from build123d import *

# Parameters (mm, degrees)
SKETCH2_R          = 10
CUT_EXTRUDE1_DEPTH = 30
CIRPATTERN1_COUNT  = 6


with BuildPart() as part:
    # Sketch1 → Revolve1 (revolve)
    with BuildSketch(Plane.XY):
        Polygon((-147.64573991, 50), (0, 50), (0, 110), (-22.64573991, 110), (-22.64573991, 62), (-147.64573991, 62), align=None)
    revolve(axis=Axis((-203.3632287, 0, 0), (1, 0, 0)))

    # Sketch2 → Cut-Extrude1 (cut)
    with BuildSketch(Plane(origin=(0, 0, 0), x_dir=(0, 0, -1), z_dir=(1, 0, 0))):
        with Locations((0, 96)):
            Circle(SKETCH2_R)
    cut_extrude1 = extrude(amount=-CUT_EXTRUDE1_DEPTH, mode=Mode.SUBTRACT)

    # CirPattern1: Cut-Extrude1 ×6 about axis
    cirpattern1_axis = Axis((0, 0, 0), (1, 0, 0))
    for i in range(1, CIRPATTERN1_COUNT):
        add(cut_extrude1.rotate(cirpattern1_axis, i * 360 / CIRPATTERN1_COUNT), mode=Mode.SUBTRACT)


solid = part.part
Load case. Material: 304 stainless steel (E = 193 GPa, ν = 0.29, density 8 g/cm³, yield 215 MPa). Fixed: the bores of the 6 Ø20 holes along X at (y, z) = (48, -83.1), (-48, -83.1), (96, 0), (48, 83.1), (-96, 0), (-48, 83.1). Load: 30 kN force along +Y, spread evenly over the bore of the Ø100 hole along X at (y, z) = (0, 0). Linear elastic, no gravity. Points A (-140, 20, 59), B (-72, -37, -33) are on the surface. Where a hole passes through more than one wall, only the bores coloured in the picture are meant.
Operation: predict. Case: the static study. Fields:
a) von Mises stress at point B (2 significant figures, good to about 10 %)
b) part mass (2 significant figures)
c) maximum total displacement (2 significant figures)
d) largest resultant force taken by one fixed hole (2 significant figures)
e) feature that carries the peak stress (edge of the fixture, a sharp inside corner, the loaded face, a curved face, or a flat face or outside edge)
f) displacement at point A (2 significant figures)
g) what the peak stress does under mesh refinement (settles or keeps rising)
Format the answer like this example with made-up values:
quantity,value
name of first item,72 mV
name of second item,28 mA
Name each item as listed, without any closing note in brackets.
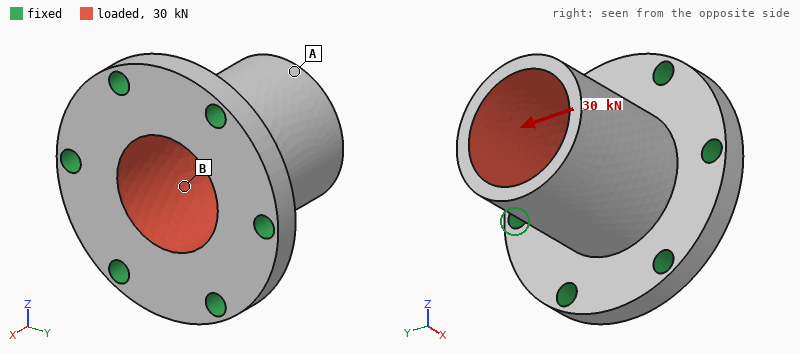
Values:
quantity,value
von Mises stress at point B,12 MPa
part mass,9.3 kg
maximum total displacement,33 µm
largest resultant force taken by one fixed hole,11 kN
feature that carries the peak stress,edge of the fixture
displacement at point A,29 µm
what the peak stress does under mesh refinement,keeps rising
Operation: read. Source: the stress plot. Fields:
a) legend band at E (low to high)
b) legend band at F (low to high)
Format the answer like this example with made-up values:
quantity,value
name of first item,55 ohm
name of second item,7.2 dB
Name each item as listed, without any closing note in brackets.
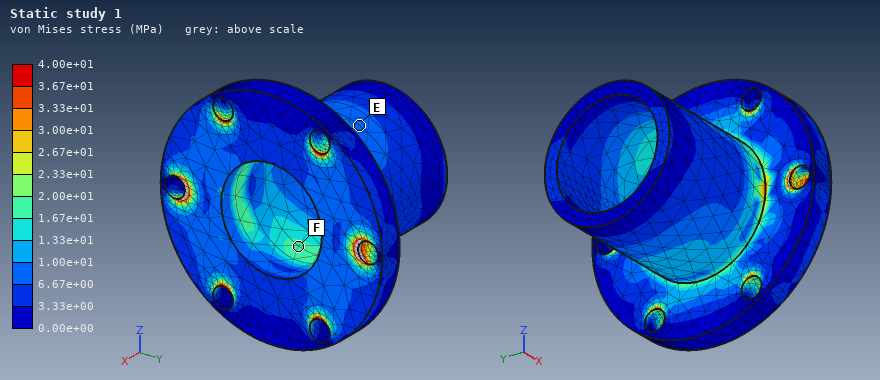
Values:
quantity,value
legend band at E,6.67e+00 to 1.00e+01 MPa
legend band at F,1.67e+01 to 2.00e+01 MPa
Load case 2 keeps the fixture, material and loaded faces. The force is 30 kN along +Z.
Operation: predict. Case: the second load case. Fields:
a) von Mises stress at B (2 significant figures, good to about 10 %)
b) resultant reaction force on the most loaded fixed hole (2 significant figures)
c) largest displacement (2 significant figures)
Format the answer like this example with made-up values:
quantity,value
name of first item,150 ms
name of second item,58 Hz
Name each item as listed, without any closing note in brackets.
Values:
quantity,value
von Mises stress at B,13 MPa
resultant reaction force on the most loaded fixed hole,9.3 kN
largest displacement,33 µm
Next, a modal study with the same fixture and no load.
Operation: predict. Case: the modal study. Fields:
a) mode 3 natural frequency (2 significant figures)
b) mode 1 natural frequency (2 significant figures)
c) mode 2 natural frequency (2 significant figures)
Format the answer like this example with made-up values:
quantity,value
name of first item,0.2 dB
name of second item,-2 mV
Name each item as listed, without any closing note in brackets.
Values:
quantity,value
mode 3 natural frequency,2900 Hz
mode 1 natural frequency,2500 Hz
mode 2 natural frequency,2500 Hz
